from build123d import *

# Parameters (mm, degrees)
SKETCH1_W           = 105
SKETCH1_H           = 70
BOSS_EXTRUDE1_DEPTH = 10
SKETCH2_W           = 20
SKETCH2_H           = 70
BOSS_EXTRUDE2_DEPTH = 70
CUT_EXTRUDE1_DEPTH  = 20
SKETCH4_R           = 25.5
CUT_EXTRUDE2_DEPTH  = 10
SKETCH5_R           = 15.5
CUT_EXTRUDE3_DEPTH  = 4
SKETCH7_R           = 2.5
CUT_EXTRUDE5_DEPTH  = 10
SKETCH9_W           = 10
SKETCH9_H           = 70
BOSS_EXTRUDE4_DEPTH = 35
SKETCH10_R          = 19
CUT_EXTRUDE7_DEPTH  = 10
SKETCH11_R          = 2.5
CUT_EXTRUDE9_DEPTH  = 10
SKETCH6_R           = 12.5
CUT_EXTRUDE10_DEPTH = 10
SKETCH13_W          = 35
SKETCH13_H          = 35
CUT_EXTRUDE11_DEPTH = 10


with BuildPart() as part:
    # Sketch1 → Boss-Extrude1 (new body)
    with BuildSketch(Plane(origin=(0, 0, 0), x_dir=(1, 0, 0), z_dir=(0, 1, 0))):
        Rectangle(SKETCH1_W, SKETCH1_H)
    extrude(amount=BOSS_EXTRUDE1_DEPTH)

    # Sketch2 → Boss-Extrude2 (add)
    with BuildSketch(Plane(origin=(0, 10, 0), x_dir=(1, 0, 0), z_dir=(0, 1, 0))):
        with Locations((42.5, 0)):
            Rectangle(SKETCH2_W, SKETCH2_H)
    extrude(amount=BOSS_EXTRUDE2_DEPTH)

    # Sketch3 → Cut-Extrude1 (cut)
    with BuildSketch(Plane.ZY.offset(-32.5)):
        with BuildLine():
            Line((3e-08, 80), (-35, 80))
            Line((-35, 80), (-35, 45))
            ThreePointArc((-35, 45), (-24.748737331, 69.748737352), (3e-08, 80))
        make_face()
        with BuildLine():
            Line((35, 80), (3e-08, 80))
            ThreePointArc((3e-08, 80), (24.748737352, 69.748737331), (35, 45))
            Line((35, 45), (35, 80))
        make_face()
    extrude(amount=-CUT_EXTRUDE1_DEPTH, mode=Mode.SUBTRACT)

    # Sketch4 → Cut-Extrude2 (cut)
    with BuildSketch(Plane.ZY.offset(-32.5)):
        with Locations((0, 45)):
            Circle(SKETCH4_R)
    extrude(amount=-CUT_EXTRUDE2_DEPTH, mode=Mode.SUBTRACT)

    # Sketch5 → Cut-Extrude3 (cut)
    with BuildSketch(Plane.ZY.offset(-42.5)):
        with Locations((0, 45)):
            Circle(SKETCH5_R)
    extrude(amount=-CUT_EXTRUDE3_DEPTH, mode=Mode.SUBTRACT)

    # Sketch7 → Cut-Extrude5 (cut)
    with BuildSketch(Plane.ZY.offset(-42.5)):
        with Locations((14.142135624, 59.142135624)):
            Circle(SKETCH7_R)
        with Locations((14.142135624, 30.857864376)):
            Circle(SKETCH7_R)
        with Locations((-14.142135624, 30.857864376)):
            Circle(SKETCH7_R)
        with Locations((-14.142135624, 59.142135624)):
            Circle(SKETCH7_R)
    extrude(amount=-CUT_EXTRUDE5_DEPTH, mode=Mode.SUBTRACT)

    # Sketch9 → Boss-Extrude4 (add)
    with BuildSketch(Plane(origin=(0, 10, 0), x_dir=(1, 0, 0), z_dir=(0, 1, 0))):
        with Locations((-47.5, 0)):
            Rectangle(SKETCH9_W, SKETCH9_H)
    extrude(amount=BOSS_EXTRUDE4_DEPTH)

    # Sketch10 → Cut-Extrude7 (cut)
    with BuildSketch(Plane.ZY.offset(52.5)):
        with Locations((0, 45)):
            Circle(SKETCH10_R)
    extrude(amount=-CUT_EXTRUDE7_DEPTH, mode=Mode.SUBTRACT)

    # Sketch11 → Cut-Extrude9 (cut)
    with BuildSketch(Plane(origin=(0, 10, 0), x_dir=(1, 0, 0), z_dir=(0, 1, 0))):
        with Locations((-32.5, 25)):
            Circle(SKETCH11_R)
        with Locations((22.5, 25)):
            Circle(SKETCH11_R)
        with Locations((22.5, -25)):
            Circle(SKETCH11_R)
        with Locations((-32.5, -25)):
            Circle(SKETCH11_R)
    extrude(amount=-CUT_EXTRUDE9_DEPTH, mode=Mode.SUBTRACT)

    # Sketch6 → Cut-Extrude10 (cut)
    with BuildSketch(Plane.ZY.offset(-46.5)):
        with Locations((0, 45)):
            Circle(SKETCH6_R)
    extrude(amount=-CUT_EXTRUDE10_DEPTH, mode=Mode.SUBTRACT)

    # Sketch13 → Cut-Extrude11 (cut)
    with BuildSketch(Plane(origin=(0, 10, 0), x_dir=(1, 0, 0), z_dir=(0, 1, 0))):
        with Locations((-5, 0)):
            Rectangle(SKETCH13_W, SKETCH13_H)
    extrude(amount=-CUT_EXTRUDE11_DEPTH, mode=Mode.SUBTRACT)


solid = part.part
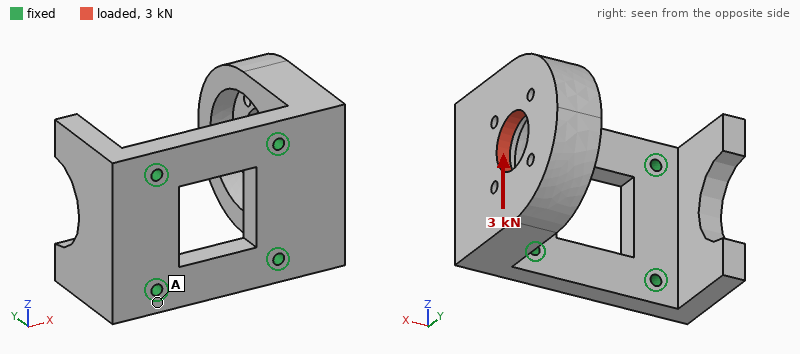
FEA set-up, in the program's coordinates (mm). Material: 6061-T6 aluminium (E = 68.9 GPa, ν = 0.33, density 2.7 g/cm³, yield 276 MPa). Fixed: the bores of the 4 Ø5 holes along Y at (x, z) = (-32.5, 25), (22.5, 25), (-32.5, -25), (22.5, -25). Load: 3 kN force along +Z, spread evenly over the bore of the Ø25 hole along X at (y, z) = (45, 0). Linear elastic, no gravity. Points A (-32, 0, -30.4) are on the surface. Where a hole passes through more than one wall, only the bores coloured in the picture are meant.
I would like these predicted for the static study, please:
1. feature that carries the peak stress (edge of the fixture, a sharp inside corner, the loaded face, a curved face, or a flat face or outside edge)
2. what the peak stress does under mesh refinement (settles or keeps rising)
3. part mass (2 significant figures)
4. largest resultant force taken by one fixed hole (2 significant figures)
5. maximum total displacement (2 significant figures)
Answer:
edge of the fixture
keeps rising
380 g
3.1 kN
68 µm
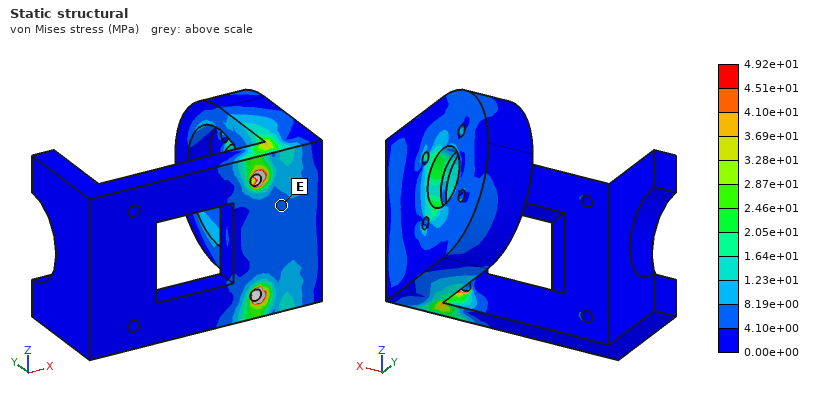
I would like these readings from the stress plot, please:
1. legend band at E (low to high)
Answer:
4.10e+00 to 8.19e+00 MPa
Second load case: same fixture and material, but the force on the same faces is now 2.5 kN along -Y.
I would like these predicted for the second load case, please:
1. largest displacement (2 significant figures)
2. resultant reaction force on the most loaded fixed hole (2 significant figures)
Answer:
0.21 mm
1.4 kN
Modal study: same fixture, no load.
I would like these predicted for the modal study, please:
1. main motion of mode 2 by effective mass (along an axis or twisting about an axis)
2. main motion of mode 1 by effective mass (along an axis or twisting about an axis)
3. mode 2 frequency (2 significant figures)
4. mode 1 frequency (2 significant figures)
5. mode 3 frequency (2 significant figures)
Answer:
along Z
along X
3000 Hz
1200 Hz
3800 Hz
